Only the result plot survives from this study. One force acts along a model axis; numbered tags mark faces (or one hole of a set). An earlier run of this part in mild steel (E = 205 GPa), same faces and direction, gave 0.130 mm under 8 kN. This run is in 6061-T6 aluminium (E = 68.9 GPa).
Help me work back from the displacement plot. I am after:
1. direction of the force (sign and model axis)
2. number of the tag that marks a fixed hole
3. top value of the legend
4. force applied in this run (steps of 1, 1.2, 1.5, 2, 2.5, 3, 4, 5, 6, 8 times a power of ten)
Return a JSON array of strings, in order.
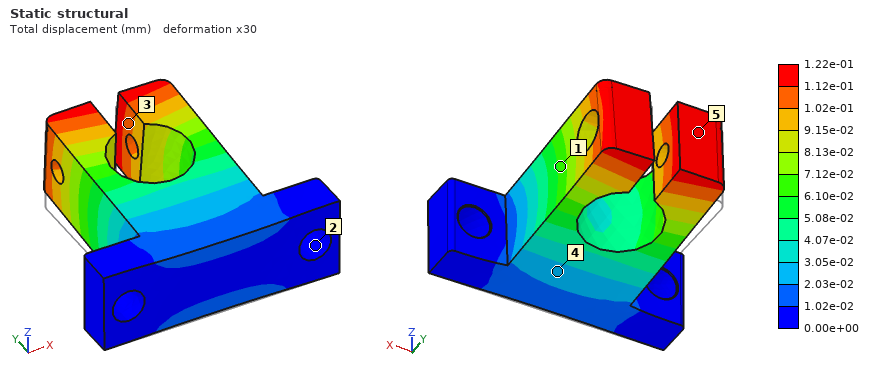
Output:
["+Z", "2", "1.22e-01 mm", "2.5 kN"]
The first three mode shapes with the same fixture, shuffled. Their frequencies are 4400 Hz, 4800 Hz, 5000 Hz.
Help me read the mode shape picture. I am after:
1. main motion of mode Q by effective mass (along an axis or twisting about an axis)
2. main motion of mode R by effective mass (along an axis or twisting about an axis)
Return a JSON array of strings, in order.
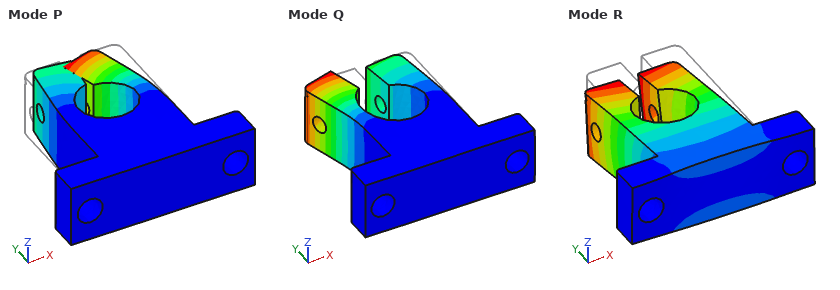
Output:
["along X", "along Z"]
